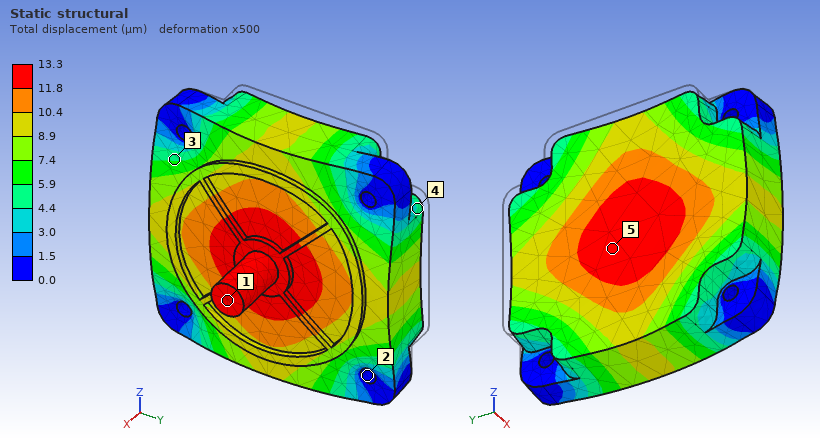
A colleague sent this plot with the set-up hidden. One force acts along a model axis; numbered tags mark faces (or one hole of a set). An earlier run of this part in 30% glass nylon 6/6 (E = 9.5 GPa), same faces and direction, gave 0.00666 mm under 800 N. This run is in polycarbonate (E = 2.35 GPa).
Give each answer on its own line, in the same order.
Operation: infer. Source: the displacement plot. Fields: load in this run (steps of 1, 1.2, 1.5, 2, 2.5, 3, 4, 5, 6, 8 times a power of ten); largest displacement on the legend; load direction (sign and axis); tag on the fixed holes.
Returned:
400 N
13.3 µm
+X
2
